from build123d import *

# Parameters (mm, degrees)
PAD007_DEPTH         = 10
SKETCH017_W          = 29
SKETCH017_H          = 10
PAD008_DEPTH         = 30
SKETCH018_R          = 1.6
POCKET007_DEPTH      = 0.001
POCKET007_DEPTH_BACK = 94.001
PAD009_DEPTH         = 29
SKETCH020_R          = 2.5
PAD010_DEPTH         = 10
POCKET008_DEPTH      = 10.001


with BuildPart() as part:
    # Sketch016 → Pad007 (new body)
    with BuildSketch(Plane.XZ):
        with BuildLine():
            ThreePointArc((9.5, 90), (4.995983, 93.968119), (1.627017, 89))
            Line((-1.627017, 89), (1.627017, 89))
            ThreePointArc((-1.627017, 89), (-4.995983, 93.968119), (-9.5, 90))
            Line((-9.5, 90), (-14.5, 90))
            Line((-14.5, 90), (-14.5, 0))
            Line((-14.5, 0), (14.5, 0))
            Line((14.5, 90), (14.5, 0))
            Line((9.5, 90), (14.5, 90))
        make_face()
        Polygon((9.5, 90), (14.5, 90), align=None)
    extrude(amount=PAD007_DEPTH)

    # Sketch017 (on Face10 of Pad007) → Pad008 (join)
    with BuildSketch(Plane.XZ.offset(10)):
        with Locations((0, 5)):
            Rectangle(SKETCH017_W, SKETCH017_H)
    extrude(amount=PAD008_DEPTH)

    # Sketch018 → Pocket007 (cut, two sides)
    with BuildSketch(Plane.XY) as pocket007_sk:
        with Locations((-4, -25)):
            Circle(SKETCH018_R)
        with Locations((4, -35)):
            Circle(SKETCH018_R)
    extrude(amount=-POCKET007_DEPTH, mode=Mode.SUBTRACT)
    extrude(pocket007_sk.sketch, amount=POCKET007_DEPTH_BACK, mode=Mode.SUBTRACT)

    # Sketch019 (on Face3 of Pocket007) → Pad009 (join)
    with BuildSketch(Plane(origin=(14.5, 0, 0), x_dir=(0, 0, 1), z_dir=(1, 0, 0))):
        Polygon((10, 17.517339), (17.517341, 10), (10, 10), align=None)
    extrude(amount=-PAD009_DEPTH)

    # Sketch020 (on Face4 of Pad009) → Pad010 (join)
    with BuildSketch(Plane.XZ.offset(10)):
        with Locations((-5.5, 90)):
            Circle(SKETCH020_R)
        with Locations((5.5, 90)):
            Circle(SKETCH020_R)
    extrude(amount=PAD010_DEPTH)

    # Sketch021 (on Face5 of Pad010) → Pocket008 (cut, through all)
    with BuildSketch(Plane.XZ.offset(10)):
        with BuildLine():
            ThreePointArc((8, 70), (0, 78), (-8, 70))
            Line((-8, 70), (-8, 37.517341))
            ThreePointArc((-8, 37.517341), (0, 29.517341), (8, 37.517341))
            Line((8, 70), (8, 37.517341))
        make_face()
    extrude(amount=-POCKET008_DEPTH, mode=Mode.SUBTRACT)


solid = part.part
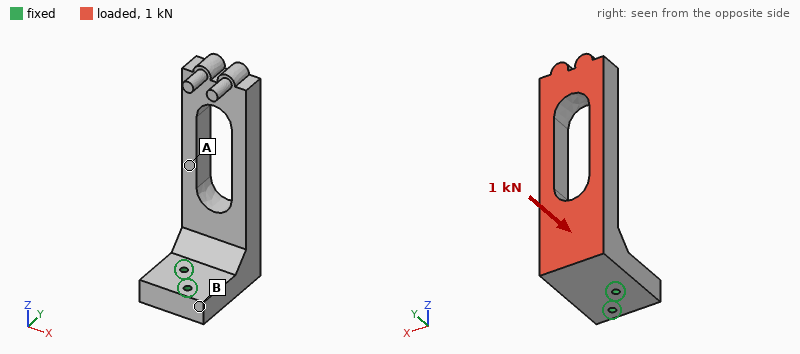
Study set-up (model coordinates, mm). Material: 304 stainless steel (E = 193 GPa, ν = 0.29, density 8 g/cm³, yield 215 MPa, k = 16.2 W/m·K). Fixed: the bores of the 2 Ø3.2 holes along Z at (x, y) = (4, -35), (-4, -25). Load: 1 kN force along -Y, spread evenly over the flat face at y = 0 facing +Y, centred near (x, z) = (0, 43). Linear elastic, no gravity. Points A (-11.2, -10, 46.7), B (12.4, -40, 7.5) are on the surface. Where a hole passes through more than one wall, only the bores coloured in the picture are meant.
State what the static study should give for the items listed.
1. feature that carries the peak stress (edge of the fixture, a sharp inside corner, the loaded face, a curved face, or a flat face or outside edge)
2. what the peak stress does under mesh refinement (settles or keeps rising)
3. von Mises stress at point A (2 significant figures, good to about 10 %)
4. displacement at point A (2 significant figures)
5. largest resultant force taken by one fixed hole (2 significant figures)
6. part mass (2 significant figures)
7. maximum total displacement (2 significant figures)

edge of the fixture
keeps rising
53 MPa
0.092 mm
1.2 kN
230 g
0.30 mm
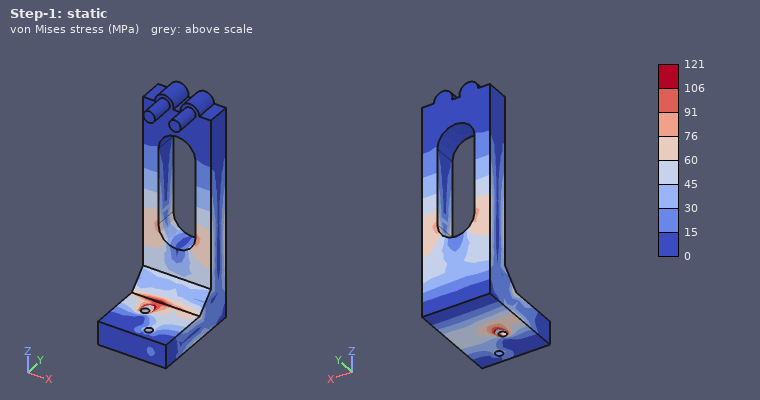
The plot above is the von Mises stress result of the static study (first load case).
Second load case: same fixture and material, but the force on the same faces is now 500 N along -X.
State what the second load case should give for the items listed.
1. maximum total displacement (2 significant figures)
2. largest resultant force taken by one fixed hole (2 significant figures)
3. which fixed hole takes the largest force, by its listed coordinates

71 µm
1.3 kN
(-4, -25)
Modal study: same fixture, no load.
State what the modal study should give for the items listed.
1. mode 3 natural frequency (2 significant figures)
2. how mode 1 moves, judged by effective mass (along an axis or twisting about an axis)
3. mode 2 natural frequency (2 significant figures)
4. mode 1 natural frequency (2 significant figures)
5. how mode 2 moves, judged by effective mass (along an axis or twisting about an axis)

3600 Hz
along Y
1200 Hz
870 Hz
along X
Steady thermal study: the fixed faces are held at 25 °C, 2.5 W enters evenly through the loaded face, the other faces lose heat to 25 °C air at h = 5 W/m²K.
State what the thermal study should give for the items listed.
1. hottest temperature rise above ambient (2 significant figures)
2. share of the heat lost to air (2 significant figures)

27 K
23 %
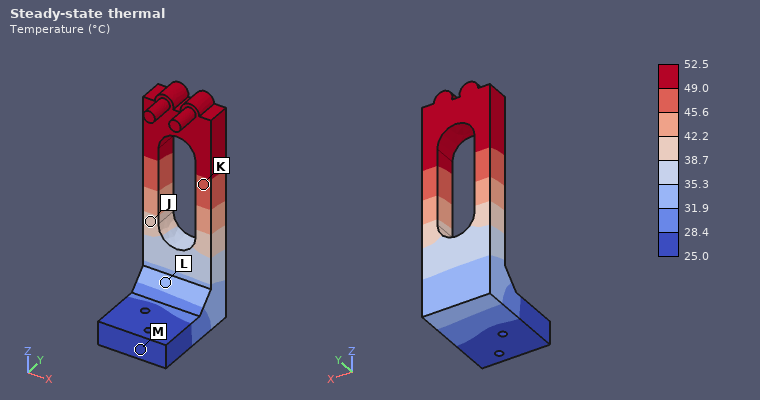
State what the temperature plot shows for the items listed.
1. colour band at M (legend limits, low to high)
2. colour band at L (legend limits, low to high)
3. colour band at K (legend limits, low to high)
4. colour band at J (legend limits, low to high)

25.0 to 28.4 °C
31.9 to 35.3 °C
45.6 to 49.0 °C
38.7 to 42.2 °C
